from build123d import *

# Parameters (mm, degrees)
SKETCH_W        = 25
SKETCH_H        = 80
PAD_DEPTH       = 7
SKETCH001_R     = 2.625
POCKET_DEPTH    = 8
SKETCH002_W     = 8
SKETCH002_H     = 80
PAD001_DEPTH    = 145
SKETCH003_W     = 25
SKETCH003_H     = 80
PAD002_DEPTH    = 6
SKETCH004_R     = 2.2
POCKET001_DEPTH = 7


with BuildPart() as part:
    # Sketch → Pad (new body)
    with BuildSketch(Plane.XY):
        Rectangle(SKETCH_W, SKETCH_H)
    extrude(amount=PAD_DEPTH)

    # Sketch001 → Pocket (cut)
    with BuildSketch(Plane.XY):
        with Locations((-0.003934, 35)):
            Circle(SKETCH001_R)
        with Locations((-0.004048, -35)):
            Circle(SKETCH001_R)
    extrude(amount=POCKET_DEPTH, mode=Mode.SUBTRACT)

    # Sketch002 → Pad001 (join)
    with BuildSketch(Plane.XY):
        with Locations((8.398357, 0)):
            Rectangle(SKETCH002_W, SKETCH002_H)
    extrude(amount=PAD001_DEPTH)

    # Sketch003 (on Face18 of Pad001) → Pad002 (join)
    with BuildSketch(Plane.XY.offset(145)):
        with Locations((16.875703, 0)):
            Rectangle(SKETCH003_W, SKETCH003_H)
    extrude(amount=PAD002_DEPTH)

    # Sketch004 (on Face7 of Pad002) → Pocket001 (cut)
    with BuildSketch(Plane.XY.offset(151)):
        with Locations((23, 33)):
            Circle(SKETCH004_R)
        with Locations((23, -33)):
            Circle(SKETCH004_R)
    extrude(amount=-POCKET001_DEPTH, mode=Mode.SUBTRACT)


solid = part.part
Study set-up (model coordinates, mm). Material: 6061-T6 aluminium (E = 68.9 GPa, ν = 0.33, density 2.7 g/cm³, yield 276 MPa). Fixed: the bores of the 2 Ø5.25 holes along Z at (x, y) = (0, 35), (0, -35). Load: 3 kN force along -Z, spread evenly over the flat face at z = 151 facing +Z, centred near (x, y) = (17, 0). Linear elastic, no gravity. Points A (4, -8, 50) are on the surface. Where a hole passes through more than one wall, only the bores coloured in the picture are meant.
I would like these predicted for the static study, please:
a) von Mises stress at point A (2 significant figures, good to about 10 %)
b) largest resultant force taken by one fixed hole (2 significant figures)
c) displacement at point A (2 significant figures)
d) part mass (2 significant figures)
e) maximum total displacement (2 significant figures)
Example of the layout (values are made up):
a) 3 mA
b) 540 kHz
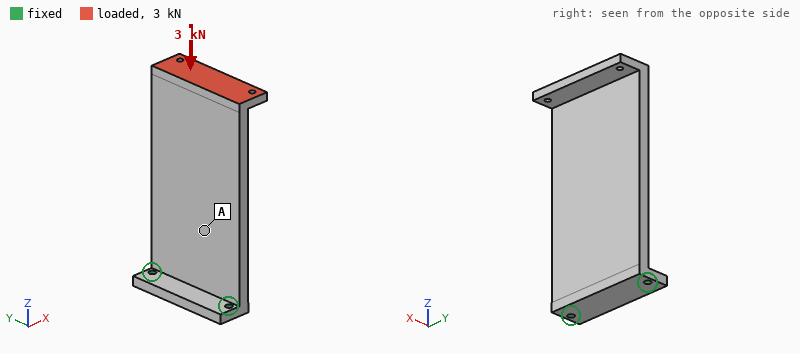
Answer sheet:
a) 25 MPa
b) 1.5 kN
c) 0.28 mm
d) 310 g
e) 1.7 mm
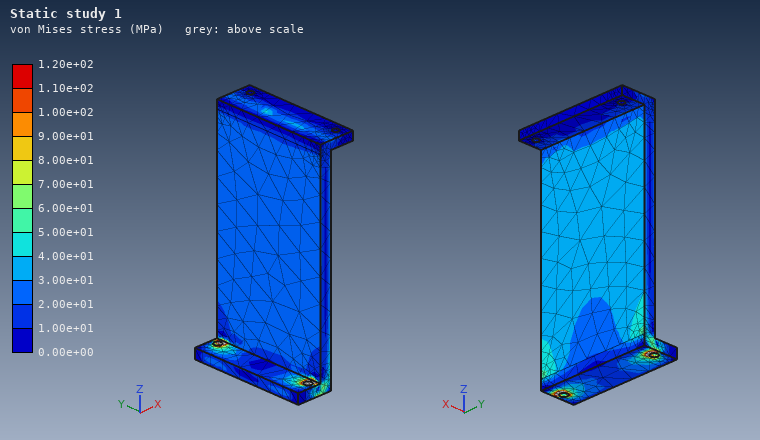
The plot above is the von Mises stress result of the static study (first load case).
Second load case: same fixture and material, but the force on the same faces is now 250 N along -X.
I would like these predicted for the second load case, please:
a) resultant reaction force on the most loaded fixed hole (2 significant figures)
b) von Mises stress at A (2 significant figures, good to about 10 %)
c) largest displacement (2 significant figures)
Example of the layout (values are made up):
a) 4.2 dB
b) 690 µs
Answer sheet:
a) 150 N
b) 29 MPa
c) 1.6 mm
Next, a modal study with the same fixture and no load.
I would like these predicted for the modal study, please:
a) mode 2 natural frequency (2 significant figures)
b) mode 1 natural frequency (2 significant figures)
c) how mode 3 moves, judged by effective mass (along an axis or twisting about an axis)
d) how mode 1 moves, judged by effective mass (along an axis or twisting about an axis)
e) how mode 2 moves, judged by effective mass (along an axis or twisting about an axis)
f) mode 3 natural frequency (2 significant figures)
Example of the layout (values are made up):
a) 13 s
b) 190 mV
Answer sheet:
a) 1000 Hz
b) 210 Hz
c) along X
d) along X
e) twisting about Z
f) 1400 Hz
